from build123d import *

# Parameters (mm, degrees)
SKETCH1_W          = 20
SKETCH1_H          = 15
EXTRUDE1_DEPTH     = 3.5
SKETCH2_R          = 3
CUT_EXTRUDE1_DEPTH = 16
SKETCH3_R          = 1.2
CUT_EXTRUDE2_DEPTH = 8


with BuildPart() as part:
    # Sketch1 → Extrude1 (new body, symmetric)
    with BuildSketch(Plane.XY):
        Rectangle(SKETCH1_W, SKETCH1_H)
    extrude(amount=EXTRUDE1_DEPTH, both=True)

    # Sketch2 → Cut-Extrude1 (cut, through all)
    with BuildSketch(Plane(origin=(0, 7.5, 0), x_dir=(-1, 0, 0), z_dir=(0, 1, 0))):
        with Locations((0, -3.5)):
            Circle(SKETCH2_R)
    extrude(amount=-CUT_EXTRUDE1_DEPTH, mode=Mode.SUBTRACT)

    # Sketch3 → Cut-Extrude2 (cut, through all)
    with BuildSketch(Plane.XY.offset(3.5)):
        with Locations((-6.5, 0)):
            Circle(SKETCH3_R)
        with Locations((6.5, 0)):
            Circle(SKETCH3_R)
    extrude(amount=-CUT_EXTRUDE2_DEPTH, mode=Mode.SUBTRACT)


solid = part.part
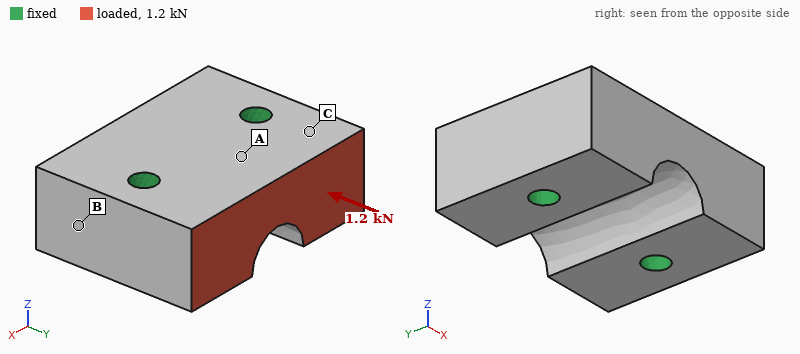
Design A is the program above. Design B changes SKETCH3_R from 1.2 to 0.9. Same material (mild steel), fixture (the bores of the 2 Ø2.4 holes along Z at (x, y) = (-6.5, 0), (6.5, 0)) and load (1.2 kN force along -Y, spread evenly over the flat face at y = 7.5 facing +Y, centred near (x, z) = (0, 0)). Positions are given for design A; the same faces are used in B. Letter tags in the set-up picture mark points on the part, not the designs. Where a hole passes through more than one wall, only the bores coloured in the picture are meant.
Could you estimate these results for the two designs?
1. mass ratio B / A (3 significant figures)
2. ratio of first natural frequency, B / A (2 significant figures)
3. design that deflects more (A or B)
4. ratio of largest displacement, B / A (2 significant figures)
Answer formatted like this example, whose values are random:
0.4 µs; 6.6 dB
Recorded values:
1.02; 0.89; B; 1.1
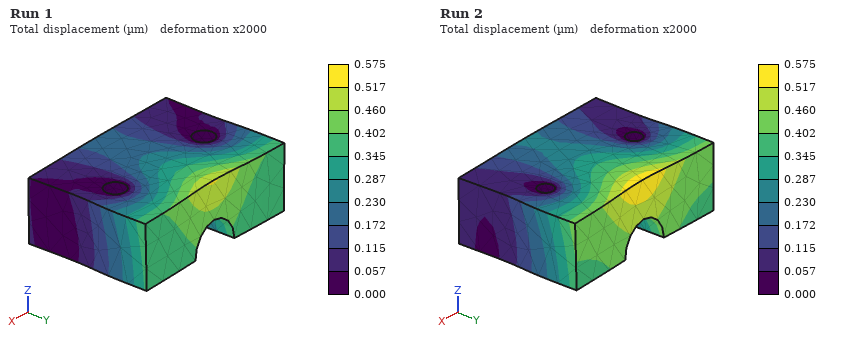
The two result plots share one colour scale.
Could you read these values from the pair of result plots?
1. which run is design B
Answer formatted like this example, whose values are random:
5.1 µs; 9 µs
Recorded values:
Run 2
